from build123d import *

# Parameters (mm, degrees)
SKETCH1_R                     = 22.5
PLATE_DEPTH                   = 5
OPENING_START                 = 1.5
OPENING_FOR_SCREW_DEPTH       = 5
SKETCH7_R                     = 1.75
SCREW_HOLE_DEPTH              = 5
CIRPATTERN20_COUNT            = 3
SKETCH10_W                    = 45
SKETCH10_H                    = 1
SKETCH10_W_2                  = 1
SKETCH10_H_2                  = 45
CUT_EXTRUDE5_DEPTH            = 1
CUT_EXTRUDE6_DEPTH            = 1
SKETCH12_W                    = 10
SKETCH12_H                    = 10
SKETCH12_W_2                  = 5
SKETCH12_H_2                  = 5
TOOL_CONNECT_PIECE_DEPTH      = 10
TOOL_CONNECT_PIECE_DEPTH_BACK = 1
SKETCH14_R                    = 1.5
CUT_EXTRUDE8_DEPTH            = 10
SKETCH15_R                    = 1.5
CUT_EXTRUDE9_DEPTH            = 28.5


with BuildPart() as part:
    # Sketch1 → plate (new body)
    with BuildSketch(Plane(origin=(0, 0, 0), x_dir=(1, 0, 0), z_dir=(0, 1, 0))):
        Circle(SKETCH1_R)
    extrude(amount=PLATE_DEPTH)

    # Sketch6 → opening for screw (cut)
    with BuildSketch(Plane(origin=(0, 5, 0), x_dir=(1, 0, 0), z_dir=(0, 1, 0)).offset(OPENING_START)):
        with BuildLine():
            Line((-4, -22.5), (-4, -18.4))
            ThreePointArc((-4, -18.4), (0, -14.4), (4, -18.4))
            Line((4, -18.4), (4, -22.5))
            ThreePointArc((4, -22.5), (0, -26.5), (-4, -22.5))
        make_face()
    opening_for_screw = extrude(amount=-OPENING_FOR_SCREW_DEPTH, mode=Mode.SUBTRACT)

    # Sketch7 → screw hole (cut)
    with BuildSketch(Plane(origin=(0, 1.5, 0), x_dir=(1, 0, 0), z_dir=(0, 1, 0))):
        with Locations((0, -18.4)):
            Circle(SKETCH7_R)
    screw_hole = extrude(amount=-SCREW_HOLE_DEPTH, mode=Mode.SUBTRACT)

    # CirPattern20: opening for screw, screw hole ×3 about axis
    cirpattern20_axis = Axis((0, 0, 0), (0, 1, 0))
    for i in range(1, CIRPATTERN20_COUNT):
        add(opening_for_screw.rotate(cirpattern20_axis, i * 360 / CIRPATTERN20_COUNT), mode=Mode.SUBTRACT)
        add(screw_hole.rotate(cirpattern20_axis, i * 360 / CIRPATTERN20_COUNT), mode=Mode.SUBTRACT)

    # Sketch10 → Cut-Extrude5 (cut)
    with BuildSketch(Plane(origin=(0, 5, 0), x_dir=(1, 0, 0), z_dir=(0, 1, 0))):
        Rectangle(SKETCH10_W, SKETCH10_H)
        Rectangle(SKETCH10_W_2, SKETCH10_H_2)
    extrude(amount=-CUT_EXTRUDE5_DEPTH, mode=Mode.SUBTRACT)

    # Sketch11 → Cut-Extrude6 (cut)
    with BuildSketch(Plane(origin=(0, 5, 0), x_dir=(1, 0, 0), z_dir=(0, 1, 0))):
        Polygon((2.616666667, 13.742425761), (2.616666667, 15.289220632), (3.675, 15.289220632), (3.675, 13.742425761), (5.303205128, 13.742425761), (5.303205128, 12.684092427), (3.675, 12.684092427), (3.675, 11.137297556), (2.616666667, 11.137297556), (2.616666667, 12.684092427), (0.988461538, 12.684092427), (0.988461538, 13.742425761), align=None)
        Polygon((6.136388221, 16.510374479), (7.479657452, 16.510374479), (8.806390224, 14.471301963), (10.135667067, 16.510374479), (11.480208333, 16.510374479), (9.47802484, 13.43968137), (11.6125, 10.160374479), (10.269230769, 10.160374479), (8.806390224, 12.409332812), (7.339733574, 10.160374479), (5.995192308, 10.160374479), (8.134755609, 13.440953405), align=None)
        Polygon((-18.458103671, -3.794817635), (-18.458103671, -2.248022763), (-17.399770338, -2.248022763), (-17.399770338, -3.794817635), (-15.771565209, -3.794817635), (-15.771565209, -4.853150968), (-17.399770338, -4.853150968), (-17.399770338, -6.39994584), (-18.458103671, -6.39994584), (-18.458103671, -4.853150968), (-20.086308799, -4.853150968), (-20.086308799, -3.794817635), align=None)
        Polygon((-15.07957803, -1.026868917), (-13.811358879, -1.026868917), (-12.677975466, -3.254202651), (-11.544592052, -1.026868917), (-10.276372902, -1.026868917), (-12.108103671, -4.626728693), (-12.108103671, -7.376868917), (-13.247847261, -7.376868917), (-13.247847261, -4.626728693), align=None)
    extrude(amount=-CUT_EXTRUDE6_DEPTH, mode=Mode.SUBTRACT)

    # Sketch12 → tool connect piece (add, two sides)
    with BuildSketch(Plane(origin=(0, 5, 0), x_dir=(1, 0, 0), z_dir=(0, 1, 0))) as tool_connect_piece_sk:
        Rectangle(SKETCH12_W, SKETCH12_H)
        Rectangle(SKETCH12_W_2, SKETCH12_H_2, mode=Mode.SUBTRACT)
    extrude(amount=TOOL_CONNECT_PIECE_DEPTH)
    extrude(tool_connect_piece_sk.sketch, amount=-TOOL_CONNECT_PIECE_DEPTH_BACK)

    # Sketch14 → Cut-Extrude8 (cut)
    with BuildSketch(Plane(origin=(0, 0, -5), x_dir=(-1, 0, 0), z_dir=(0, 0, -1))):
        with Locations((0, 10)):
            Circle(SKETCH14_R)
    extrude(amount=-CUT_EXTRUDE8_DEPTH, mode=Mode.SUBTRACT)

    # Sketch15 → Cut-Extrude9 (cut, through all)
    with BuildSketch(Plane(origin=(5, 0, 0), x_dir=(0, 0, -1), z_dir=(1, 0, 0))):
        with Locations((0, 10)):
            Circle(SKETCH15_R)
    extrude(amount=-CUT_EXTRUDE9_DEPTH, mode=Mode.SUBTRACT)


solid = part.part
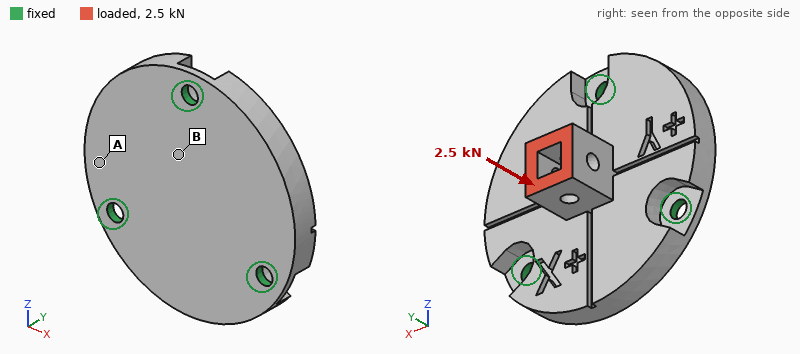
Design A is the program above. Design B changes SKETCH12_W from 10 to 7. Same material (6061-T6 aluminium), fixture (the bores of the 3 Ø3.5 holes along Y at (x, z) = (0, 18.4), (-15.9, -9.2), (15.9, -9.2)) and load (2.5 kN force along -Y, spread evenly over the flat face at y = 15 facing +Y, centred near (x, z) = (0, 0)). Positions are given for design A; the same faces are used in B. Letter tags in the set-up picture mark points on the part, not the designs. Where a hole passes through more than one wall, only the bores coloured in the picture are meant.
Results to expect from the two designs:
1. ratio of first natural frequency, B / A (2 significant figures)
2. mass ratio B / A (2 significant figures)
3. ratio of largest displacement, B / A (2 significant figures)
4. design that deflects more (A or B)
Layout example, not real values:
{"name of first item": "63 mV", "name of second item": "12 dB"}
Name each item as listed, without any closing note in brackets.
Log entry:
{"ratio of first natural frequency, B / A": "0.99", "mass ratio B / A": "0.96", "ratio of largest displacement, B / A": "1.2", "design that deflects more": "B"}
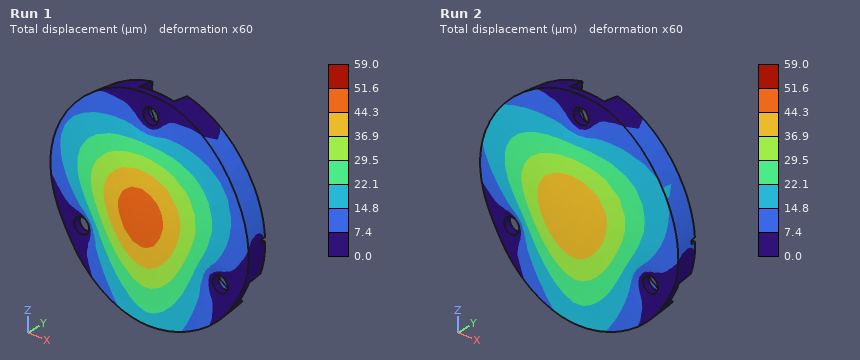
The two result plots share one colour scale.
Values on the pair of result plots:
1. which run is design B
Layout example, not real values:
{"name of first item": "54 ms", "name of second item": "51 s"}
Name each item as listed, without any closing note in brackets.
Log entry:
{"which run is design B": "Run 1"}
